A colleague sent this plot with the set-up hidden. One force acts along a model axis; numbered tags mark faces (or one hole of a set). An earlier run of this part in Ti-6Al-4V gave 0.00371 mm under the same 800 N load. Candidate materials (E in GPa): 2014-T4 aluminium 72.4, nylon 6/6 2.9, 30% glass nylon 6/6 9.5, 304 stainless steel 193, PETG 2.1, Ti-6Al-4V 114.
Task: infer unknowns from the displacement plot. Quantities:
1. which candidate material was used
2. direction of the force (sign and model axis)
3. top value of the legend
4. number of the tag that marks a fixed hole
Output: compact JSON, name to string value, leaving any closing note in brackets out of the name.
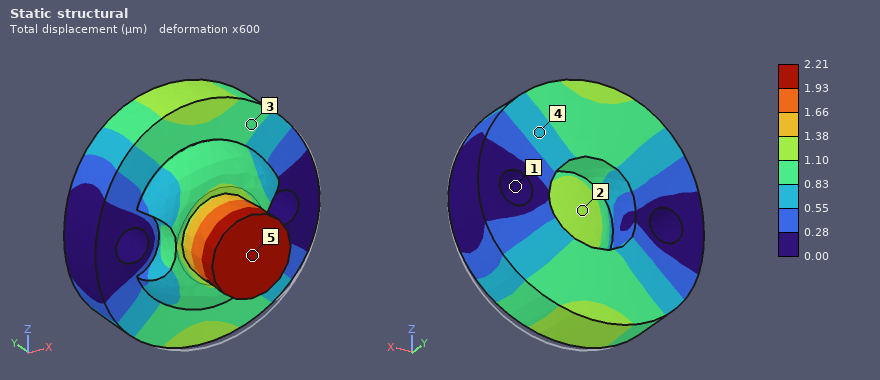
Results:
{"which candidate material was used": "304 stainless steel", "direction of the force": "+Y", "top value of the legend": "2.21 µm", "number of the tag that marks a fixed hole": "1"}
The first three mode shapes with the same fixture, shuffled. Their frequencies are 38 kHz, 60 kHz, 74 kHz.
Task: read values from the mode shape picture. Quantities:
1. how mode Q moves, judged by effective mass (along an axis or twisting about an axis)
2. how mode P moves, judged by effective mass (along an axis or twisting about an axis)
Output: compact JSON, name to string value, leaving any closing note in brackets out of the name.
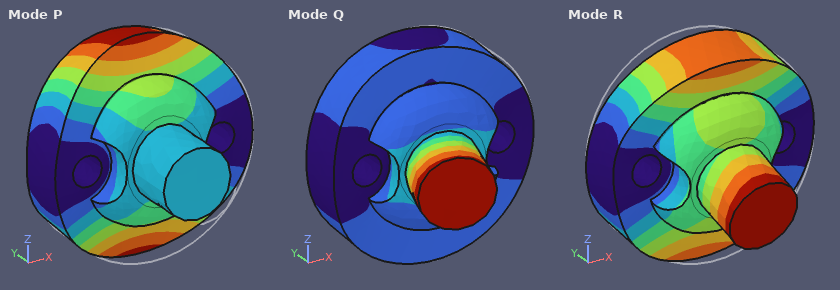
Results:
{"how mode Q moves, judged by effective mass": "along X", "how mode P moves, judged by effective mass": "along Y"}
